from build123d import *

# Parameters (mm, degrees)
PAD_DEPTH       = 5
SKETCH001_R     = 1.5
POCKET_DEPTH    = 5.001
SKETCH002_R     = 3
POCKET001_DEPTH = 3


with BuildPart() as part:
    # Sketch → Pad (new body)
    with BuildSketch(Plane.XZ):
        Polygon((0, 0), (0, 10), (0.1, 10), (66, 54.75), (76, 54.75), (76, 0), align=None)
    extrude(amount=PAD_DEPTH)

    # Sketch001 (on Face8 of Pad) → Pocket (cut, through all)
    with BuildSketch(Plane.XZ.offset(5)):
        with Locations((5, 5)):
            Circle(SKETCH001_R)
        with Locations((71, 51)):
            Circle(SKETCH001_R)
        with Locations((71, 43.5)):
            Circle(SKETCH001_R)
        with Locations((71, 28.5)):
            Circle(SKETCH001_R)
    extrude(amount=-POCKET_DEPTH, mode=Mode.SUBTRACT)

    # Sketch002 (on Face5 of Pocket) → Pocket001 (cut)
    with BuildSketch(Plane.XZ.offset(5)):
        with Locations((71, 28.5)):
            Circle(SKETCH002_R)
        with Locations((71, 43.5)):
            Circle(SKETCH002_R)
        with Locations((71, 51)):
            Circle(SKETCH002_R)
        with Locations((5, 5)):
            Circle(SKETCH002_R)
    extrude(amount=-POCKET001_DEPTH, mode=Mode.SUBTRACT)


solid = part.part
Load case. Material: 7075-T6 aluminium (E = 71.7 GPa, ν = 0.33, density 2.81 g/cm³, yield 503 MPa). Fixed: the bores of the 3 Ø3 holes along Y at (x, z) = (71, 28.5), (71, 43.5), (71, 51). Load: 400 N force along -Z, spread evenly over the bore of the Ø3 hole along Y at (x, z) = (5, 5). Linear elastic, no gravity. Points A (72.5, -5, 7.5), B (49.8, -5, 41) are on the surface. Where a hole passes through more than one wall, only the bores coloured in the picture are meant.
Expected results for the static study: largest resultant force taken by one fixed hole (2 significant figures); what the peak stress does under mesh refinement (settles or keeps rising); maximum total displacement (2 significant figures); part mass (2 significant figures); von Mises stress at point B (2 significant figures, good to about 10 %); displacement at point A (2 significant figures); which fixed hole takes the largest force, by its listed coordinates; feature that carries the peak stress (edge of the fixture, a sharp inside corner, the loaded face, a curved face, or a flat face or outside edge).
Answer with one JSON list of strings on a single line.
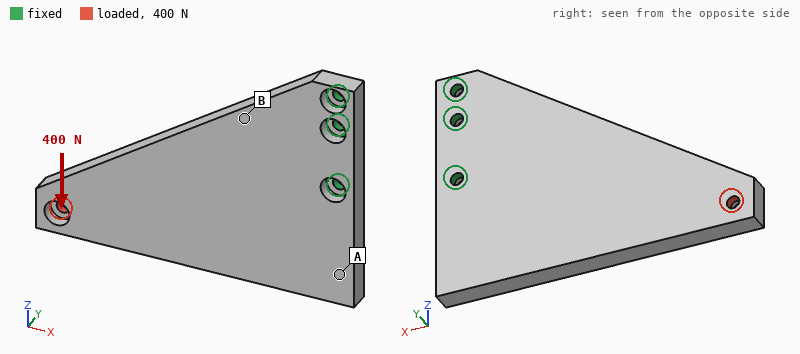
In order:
["1.2 kN", "keeps rising", "0.13 mm", "37 g", "16 MPa", "0.033 mm", "(71, 28.5)", "edge of the fixture"]
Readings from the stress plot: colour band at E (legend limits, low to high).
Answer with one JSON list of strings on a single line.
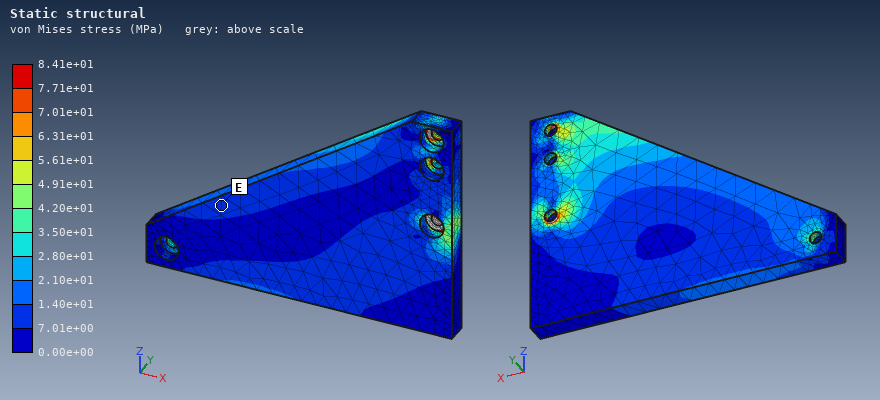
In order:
["7.01e+00 to 1.40e+01 MPa"]
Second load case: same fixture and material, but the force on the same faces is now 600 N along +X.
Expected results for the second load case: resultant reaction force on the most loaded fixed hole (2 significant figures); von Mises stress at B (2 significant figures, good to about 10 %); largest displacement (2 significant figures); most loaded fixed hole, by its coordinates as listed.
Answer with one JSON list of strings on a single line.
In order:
["1.2 kN", "13 MPa", "91 µm", "(71, 28.5)"]
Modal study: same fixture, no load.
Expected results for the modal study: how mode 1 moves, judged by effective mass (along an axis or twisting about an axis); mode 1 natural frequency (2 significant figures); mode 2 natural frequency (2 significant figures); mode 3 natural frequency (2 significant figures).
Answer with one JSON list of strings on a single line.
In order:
["along Y", "740 Hz", "3100 Hz", "3900 Hz"]
